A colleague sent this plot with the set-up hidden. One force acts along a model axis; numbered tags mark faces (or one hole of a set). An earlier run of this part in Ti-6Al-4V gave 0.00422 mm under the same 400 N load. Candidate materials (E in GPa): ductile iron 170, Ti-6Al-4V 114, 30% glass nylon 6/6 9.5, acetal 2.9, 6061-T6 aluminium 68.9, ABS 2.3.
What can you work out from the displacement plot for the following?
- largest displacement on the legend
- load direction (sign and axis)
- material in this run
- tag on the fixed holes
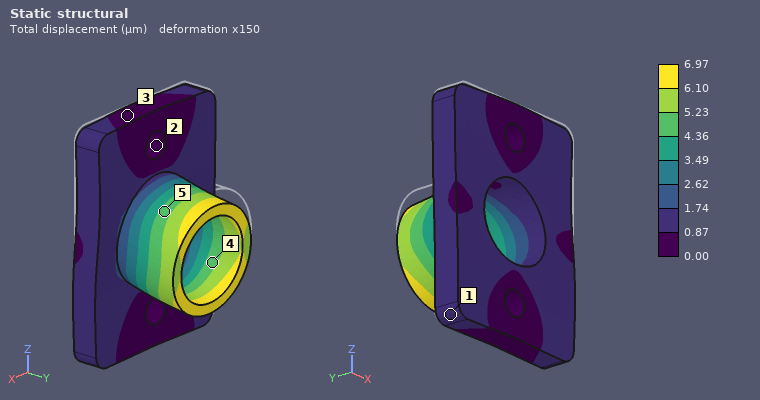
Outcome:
6.97 µm
-Z
6061-T6 aluminium
2
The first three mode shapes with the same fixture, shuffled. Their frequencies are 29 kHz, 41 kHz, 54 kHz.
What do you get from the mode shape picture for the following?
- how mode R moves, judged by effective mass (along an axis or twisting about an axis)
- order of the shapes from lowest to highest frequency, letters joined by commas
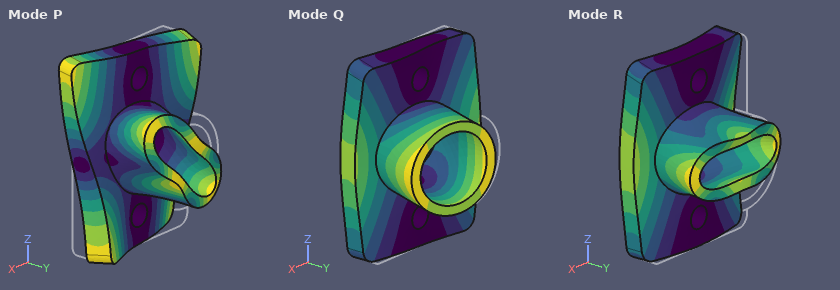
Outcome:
along Y
Q, R, P
